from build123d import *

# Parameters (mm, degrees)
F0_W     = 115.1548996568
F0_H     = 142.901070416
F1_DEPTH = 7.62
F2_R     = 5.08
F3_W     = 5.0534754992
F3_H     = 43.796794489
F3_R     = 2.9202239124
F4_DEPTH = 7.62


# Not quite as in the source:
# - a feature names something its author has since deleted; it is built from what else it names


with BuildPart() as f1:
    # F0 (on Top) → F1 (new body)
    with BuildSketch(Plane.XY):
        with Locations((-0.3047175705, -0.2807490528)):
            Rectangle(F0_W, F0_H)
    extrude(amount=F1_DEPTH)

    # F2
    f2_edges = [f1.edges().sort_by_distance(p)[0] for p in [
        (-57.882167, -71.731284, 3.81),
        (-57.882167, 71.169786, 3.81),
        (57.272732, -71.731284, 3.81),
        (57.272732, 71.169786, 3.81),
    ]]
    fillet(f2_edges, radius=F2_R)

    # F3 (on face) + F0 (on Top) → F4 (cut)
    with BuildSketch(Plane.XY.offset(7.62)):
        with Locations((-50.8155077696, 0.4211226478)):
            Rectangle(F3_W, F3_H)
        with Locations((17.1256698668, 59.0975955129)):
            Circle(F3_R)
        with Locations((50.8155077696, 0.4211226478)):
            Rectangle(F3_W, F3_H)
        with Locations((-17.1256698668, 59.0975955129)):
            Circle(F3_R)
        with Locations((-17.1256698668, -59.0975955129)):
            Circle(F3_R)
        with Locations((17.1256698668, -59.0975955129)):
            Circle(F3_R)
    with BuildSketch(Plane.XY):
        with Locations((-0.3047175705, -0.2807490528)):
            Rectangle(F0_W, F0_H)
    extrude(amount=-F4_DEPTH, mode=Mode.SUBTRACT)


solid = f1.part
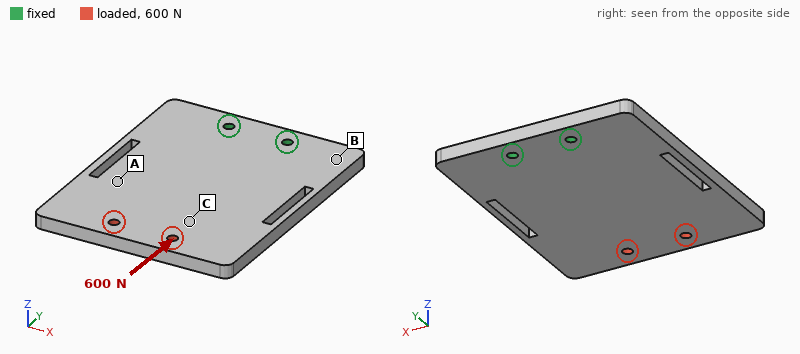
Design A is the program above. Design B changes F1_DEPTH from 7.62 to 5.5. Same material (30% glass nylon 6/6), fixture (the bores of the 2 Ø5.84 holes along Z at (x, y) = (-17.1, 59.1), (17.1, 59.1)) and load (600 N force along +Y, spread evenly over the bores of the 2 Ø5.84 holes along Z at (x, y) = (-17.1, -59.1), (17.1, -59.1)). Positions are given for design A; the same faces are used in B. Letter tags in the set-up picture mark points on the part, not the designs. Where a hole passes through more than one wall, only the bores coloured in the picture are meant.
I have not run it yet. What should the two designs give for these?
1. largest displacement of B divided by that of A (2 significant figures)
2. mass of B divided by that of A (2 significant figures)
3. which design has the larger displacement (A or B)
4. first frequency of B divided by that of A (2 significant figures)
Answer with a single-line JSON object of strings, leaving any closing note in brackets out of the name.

{"largest displacement of B divided by that of A": "1.4", "mass of B divided by that of A": "0.72", "which design has the larger displacement": "B", "first frequency of B divided by that of A": "0.74"}
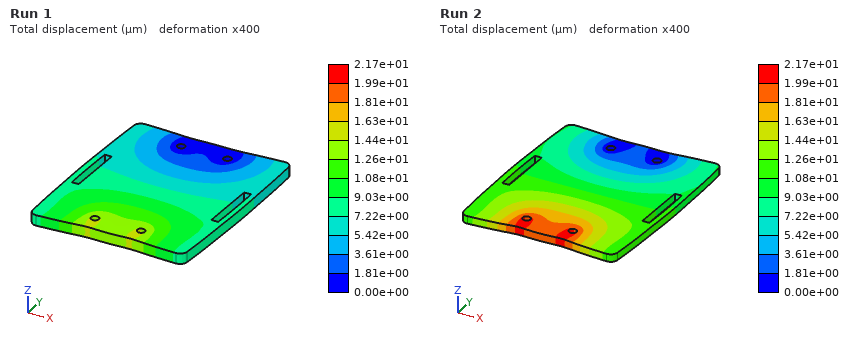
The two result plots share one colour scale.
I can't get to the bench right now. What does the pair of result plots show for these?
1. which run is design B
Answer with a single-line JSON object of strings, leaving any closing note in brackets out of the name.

{"which run is design B": "Run 2"}
